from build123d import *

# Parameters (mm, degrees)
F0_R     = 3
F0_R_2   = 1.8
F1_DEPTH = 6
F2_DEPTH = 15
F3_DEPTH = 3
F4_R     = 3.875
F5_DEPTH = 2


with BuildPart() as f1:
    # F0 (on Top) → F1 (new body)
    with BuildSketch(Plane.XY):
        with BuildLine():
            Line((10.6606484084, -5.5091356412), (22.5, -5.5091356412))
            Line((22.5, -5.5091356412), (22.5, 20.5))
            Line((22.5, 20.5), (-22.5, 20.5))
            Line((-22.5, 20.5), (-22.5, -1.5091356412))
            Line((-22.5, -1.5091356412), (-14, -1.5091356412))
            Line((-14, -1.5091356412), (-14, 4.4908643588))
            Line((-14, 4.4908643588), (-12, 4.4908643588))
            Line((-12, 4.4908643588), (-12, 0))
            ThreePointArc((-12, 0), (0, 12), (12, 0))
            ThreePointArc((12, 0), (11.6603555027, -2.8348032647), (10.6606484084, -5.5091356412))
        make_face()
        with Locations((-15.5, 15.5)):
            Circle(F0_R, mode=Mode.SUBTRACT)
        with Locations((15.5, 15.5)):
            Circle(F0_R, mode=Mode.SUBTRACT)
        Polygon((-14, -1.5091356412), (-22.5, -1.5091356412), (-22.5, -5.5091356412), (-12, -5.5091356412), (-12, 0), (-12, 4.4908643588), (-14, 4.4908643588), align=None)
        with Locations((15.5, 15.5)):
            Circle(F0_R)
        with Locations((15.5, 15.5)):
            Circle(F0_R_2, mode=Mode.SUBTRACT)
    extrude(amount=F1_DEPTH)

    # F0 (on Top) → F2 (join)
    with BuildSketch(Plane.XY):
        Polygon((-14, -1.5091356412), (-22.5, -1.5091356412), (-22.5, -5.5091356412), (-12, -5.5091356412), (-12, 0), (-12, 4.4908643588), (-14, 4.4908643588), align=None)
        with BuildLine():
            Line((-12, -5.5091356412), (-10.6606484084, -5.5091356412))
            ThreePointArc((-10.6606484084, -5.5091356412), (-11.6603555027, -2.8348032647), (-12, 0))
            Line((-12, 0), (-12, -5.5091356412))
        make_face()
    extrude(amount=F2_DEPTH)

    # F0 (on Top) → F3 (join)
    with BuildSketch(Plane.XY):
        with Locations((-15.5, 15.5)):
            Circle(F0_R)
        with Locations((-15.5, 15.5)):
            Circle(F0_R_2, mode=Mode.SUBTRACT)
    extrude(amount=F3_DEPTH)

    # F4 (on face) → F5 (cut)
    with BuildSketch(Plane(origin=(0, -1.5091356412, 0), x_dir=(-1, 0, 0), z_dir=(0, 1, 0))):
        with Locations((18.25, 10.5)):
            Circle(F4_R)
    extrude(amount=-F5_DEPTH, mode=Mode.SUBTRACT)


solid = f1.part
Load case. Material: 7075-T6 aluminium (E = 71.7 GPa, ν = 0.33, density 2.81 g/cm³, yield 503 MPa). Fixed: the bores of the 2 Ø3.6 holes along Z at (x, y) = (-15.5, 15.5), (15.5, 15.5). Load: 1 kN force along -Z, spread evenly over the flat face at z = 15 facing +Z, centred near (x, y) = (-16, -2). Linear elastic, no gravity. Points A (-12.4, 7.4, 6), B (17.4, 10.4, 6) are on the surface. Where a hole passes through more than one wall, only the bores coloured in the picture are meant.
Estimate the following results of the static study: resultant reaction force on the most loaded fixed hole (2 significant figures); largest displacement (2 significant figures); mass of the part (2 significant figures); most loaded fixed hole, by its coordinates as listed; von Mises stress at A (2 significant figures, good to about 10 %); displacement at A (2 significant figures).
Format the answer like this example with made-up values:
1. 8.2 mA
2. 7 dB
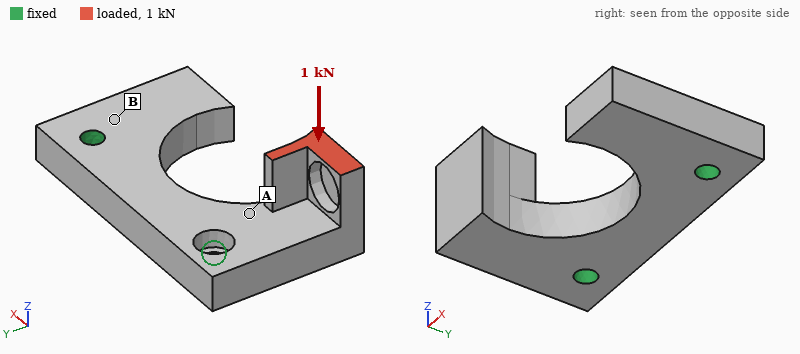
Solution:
1. 1.1 kN
2. 0.34 mm
3. 14 g
4. (-15.5, 15.5)
5. 140 MPa
6. 0.087 mm
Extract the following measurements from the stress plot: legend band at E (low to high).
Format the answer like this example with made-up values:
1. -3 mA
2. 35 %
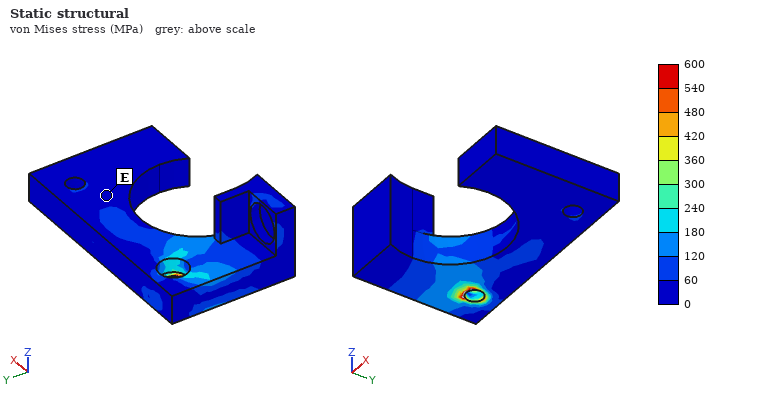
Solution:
1. 0 to 60 MPa
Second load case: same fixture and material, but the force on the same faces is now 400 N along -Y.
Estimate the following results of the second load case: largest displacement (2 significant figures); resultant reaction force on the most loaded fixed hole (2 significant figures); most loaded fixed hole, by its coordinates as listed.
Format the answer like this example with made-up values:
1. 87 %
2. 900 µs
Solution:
1. 0.16 mm
2. 370 N
3. (-15.5, 15.5)
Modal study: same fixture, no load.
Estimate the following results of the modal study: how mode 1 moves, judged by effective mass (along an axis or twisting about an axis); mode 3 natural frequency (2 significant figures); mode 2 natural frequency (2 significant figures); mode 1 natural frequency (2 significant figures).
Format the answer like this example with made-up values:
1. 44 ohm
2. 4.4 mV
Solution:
1. along Z
2. 12 kHz
3. 10 kHz
4. 5800 Hz
